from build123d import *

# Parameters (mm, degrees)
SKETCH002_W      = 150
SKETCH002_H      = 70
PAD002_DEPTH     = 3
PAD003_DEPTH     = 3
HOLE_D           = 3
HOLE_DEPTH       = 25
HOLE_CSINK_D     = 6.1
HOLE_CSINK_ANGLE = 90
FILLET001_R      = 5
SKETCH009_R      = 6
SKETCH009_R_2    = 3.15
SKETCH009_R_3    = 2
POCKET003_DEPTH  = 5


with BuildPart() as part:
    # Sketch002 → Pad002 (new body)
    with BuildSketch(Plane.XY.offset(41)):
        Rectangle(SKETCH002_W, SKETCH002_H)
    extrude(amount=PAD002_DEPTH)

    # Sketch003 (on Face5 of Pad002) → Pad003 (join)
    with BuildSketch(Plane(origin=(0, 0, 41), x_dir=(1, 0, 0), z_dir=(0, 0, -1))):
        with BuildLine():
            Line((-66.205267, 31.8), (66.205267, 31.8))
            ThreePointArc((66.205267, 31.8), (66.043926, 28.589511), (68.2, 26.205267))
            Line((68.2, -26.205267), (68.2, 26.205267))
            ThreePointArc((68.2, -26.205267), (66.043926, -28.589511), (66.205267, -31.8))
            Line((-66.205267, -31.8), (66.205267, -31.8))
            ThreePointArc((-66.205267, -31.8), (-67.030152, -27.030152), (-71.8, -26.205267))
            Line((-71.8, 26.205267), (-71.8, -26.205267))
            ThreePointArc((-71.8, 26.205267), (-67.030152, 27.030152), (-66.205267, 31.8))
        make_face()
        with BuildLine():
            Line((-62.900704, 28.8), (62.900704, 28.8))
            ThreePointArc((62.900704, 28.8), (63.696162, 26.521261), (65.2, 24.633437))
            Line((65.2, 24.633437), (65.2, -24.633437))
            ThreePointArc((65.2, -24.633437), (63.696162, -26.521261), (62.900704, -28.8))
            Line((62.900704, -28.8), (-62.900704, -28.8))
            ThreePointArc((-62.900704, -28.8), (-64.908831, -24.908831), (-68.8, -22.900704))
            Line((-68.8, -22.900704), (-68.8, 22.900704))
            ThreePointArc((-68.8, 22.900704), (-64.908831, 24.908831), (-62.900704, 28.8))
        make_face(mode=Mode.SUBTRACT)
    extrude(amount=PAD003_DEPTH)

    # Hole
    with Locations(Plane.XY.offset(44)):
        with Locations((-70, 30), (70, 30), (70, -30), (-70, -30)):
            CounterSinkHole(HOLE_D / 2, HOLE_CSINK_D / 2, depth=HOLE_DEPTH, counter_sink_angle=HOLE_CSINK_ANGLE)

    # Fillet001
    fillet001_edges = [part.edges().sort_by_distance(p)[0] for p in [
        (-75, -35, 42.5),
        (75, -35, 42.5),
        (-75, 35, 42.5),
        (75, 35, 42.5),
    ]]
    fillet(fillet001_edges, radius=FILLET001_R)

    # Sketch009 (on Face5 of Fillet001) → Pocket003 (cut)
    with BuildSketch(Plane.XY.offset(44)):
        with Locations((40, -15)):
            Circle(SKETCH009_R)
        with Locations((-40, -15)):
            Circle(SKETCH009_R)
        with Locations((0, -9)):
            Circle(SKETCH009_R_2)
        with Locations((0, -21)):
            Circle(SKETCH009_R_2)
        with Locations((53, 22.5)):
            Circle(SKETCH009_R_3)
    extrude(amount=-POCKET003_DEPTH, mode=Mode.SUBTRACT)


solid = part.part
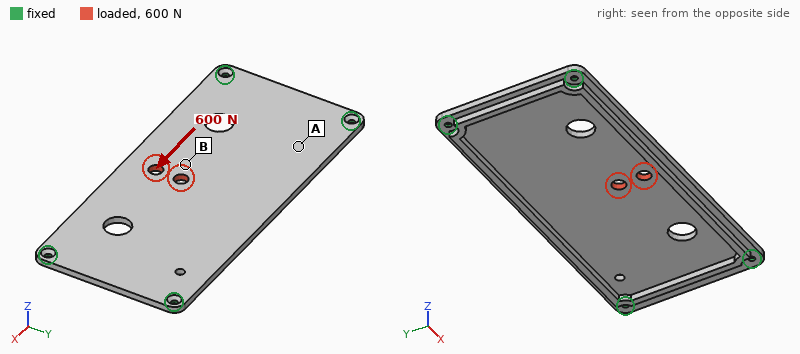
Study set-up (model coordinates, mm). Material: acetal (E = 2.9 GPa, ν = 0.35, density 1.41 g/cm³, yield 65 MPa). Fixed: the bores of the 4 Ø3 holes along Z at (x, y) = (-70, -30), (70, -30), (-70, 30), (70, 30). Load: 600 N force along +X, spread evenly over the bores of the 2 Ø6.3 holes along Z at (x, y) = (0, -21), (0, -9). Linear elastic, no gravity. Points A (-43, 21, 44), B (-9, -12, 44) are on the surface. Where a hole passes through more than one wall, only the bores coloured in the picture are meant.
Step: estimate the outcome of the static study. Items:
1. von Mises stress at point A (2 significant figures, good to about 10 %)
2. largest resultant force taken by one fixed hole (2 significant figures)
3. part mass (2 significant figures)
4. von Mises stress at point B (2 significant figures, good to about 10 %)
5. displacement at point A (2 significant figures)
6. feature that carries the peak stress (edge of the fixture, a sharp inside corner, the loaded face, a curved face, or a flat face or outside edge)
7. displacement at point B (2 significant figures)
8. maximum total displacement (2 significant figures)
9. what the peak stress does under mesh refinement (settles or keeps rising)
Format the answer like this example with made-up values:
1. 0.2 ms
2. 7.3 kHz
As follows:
1. 1.4 MPa
2. 170 N
3. 48 g
4. 3.7 MPa
5. 30 µm
6. edge of the fixture
7. 69 µm
8. 82 µm
9. keeps rising
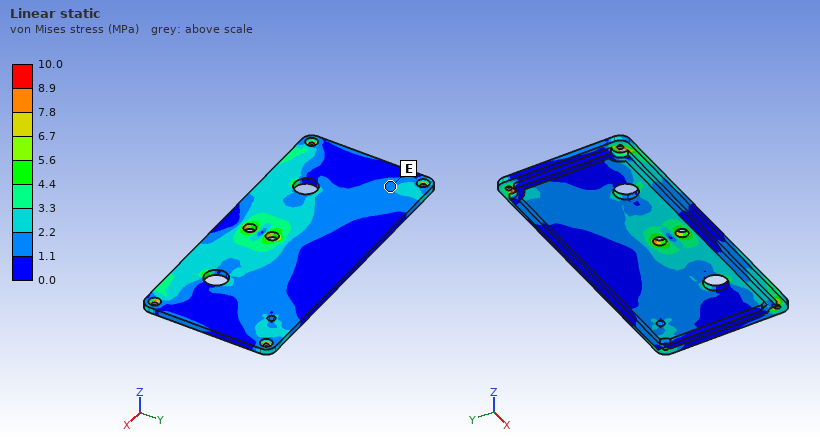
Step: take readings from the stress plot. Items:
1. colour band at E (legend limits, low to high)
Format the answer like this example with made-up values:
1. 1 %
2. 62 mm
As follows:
1. 1.1 to 2.2 MPa
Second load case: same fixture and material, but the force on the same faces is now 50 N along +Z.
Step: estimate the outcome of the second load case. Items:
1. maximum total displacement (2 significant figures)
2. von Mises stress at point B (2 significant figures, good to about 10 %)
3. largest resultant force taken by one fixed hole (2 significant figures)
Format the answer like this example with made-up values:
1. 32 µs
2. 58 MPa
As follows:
1. 2.0 mm
2. 5.6 MPa
3. 24 N
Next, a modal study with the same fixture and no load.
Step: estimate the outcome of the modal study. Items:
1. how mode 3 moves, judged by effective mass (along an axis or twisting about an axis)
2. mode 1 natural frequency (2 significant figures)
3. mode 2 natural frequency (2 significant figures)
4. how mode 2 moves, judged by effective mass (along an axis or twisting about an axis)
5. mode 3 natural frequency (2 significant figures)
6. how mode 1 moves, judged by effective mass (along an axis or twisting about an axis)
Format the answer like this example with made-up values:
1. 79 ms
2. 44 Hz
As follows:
1. twisting about Y
2. 210 Hz
3. 380 Hz
4. twisting about X
5. 610 Hz
6. along Z
